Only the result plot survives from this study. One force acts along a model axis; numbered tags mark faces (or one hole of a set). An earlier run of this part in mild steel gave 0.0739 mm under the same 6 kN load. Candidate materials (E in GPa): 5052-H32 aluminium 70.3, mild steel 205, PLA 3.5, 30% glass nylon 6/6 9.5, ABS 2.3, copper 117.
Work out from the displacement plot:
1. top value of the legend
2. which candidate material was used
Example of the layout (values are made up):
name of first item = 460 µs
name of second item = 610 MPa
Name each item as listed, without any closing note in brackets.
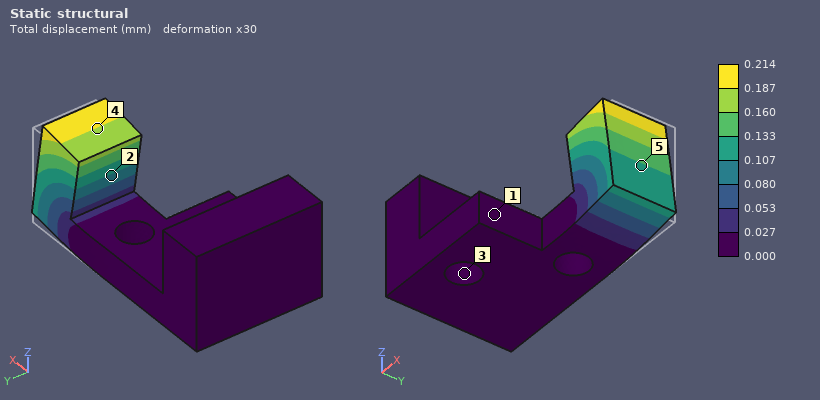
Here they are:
top value of the legend = 0.214 mm
which candidate material was used = 5052-H32 aluminium
